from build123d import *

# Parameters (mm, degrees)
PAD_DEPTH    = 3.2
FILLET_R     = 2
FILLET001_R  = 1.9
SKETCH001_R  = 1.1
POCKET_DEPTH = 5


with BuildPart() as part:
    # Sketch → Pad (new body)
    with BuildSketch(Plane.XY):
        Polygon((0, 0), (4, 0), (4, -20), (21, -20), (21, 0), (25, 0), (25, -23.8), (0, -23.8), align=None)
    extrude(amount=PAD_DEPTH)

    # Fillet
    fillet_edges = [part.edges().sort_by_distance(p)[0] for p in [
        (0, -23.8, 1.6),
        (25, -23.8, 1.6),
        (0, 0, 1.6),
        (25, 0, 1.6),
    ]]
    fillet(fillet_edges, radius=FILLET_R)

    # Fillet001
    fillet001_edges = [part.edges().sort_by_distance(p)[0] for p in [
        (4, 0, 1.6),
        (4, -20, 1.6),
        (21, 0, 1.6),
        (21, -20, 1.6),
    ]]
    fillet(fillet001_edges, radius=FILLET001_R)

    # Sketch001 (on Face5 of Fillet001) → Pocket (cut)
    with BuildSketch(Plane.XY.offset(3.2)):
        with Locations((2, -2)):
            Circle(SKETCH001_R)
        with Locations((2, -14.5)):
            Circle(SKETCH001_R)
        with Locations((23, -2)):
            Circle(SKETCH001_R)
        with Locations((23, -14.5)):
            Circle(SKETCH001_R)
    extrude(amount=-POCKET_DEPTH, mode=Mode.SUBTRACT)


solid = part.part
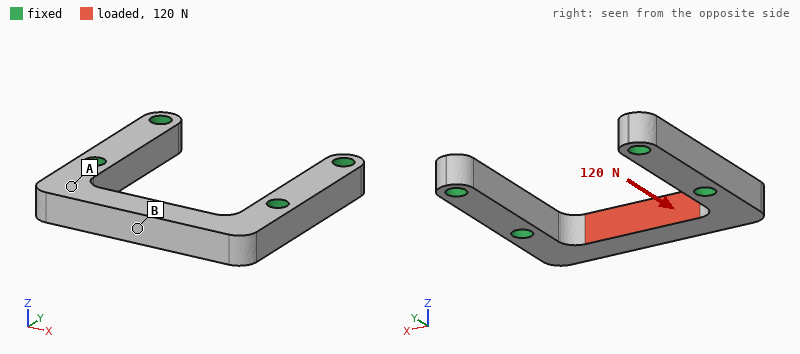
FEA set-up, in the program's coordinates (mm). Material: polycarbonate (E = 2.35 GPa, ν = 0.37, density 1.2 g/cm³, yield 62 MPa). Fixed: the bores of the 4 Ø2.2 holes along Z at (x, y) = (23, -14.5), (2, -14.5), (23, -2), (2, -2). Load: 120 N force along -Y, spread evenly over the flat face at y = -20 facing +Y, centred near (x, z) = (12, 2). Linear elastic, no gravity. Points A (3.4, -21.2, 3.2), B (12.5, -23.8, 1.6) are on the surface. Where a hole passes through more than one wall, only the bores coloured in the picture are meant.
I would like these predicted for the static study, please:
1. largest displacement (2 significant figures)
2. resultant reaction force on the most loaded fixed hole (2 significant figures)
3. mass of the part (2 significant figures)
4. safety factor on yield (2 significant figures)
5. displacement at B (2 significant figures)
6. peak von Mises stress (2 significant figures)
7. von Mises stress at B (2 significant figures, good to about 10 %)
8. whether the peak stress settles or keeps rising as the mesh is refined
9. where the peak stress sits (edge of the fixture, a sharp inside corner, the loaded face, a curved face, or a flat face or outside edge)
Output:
0.16 mm
75 N
0.91 g
1.8
0.15 mm
35 MPa
24 MPa
settles
a curved face
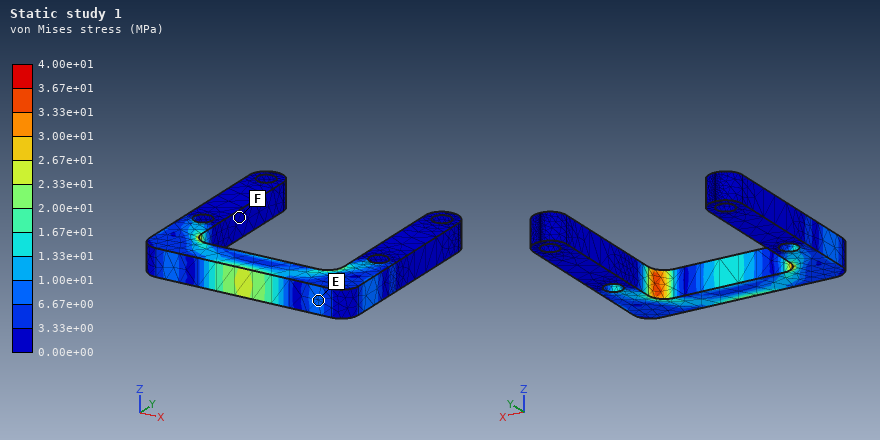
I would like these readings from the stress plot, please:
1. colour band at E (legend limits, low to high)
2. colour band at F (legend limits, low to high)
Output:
6.67e+00 to 1.00e+01 MPa
0.00e+00 to 3.33e+00 MPa
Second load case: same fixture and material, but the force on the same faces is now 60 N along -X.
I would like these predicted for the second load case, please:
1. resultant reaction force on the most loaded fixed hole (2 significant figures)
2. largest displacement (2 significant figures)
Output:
31 N
72 µm
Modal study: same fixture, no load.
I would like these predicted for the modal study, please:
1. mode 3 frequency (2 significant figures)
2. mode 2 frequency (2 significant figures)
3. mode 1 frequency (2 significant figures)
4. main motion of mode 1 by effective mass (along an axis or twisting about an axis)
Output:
8500 Hz
8300 Hz
4400 Hz
along Z
